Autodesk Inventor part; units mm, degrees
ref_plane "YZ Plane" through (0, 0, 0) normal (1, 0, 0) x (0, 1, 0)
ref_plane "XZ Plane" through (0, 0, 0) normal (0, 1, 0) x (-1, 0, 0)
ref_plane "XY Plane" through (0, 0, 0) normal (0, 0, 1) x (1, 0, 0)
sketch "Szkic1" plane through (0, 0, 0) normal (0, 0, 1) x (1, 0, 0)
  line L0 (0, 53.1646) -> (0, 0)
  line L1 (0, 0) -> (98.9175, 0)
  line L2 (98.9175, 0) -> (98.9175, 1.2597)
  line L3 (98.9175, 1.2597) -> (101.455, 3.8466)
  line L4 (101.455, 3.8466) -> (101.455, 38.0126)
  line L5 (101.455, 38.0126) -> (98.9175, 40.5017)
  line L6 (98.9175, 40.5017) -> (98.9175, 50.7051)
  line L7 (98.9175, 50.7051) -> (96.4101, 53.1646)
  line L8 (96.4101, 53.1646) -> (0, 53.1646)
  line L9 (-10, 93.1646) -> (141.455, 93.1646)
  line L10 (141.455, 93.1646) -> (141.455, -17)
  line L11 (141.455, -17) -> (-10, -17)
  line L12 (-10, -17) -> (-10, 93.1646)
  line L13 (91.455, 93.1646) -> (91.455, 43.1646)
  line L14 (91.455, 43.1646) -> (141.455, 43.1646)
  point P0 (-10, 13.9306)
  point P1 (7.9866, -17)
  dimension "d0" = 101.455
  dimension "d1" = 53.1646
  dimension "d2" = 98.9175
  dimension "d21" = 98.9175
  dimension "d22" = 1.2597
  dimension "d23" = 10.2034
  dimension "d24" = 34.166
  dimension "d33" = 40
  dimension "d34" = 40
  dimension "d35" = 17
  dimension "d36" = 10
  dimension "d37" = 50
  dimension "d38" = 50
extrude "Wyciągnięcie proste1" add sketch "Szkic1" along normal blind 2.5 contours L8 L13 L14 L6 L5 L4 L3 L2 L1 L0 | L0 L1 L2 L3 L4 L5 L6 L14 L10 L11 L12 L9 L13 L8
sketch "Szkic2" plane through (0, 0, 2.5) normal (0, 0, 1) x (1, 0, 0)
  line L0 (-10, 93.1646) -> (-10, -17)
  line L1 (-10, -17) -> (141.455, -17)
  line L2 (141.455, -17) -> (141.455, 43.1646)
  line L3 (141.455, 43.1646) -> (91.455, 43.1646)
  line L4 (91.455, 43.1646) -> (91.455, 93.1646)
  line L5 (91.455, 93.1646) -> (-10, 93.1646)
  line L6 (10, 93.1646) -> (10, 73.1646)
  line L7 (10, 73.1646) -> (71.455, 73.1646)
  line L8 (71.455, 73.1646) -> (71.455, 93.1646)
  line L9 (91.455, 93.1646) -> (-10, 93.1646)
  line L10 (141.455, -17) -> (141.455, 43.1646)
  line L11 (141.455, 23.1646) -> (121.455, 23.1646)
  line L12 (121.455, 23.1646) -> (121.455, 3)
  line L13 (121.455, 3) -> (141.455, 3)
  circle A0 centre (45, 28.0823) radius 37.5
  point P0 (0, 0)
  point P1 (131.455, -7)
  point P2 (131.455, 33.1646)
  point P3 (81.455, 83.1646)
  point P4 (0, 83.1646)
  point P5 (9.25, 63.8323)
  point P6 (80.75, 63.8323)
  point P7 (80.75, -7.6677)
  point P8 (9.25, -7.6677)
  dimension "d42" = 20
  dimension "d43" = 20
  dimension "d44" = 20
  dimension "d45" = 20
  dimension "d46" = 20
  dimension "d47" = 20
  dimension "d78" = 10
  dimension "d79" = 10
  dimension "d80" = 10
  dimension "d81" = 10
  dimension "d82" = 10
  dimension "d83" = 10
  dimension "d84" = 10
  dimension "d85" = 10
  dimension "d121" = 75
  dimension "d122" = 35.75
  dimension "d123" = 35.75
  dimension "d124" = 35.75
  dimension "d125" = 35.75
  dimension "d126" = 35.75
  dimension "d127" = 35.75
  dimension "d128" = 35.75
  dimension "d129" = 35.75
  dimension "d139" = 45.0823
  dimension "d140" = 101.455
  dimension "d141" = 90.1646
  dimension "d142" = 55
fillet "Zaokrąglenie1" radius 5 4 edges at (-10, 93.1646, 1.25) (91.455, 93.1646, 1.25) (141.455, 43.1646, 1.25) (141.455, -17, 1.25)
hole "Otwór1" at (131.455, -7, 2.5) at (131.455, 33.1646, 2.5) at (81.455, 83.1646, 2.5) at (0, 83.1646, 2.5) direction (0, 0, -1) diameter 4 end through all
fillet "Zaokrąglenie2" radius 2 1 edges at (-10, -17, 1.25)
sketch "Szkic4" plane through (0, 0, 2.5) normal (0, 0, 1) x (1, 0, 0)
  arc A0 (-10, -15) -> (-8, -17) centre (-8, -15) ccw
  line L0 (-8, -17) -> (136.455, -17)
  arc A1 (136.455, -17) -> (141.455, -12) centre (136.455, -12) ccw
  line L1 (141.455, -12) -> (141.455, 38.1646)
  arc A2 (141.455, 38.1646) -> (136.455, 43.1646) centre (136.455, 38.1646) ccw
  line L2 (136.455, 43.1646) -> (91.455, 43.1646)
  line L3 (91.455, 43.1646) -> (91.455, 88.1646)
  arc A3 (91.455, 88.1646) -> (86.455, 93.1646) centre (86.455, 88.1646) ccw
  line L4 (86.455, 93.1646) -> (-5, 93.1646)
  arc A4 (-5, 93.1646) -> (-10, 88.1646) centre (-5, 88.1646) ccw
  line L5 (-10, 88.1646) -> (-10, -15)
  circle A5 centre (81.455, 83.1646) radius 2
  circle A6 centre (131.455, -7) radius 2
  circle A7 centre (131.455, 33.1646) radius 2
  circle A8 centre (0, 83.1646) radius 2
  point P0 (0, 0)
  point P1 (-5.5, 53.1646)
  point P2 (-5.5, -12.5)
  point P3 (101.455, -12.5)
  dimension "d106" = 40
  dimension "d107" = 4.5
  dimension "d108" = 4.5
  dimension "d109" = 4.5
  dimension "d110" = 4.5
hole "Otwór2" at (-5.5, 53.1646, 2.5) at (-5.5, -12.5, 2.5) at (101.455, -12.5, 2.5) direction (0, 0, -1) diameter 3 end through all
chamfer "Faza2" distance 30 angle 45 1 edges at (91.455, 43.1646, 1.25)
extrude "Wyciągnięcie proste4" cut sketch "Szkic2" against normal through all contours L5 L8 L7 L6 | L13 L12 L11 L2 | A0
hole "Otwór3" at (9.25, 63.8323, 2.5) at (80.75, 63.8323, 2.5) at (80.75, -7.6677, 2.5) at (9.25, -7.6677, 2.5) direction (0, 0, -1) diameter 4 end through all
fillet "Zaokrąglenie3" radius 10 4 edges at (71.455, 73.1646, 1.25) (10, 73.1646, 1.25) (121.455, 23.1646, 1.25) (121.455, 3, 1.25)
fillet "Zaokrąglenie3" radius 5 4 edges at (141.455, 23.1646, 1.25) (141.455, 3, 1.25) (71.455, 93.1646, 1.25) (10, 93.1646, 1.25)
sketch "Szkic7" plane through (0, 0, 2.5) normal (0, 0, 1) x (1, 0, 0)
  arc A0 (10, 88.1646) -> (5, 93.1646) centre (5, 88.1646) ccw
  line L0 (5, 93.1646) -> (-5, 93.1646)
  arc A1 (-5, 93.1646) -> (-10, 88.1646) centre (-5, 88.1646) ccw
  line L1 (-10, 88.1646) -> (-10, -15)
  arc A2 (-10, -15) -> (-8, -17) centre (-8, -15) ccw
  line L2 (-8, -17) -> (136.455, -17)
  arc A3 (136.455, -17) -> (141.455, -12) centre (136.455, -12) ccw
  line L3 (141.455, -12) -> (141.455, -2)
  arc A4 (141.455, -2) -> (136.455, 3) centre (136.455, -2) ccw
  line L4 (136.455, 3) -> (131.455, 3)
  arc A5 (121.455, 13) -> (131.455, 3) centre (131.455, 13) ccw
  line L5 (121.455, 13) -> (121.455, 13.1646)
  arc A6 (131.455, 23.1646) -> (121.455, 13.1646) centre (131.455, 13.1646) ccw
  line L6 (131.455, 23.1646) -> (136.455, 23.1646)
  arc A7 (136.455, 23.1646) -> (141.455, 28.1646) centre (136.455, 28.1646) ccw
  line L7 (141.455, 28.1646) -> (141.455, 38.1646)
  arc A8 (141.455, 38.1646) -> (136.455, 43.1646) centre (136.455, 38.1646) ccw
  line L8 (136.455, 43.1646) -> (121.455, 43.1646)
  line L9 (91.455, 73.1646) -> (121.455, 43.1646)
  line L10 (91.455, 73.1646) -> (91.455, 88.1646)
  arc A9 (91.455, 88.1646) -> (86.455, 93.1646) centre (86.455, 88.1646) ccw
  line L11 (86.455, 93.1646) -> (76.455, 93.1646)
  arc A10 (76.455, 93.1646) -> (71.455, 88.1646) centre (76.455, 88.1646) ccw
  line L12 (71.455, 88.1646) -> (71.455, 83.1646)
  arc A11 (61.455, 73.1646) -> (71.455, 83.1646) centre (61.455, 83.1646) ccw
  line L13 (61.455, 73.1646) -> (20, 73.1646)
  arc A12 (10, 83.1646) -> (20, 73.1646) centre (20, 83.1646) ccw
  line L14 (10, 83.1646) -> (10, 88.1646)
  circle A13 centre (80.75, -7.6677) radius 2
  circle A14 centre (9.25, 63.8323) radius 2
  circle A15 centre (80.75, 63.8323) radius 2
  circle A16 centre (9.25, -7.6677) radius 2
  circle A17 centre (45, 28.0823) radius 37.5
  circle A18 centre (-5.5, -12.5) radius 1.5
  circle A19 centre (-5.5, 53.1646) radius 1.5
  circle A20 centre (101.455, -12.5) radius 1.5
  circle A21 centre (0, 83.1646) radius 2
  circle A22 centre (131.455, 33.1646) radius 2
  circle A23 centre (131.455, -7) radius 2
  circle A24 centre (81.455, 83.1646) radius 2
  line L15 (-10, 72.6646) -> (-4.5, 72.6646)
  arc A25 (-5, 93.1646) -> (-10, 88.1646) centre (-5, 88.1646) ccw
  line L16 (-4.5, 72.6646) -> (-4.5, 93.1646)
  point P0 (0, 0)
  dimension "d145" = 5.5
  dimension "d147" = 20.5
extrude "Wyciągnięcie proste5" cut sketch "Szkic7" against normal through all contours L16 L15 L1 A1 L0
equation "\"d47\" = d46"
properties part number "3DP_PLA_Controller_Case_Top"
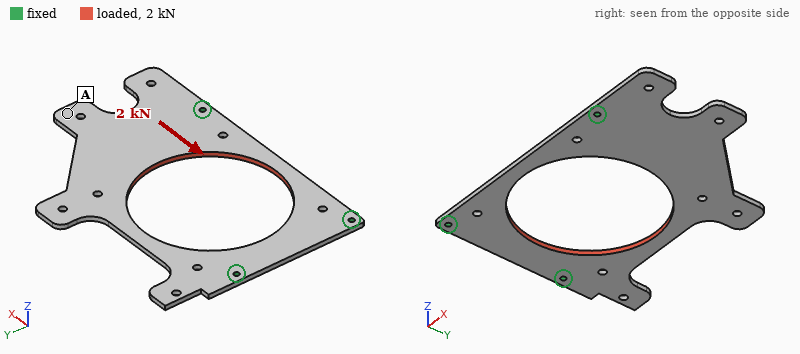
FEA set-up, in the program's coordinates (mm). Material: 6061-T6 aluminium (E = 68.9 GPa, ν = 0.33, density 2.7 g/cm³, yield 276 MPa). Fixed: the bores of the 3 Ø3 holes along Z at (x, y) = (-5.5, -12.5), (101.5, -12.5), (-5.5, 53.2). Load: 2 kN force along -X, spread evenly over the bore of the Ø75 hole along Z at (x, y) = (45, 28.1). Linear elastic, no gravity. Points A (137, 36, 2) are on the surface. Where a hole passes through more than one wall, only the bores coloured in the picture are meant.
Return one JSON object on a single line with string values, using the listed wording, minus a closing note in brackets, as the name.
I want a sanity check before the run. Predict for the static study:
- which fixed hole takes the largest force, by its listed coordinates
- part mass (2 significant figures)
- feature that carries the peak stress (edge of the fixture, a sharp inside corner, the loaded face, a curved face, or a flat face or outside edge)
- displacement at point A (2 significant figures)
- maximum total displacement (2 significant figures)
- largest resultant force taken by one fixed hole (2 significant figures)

{"which fixed hole takes the largest force, by its listed coordinates": "(-5.5, 53.2)", "part mass": "57 g", "feature that carries the peak stress": "edge of the fixture", "displacement at point A": "35 µm", "maximum total displacement": "38 µm", "largest resultant force taken by one fixed hole": "1.0 kN"}
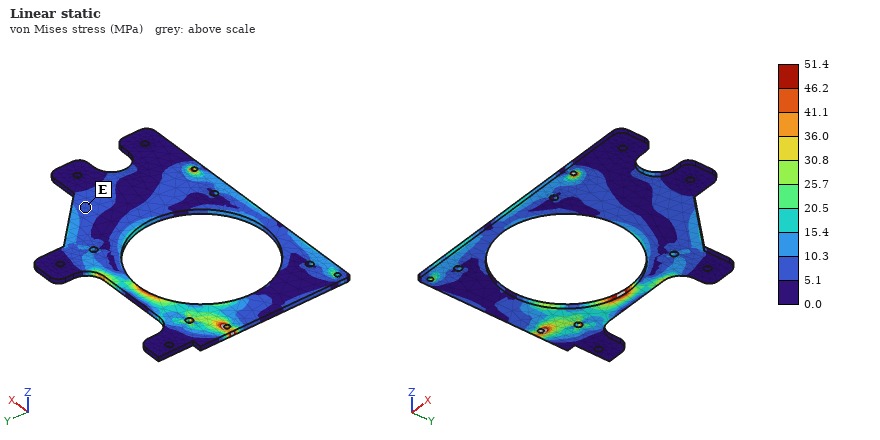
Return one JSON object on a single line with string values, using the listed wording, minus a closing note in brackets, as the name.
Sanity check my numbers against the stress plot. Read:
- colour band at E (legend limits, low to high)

{"colour band at E": "5.1 to 10.3 MPa"}
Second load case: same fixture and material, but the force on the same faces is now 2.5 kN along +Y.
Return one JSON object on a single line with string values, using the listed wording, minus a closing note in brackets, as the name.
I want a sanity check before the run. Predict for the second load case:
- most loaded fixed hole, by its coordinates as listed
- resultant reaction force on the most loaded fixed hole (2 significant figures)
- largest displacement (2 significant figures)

{"most loaded fixed hole, by its coordinates as listed": "(101.5, -12.5)", "resultant reaction force on the most loaded fixed hole": "1.3 kN", "largest displacement": "47 µm"}
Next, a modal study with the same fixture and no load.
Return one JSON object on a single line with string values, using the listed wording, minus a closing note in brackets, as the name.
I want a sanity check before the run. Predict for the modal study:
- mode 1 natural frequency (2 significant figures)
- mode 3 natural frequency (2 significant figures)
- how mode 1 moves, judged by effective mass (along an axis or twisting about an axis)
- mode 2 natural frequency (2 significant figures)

{"mode 1 natural frequency": "300 Hz", "mode 3 natural frequency": "1200 Hz", "how mode 1 moves, judged by effective mass": "along Z", "mode 2 natural frequency": "740 Hz"}
